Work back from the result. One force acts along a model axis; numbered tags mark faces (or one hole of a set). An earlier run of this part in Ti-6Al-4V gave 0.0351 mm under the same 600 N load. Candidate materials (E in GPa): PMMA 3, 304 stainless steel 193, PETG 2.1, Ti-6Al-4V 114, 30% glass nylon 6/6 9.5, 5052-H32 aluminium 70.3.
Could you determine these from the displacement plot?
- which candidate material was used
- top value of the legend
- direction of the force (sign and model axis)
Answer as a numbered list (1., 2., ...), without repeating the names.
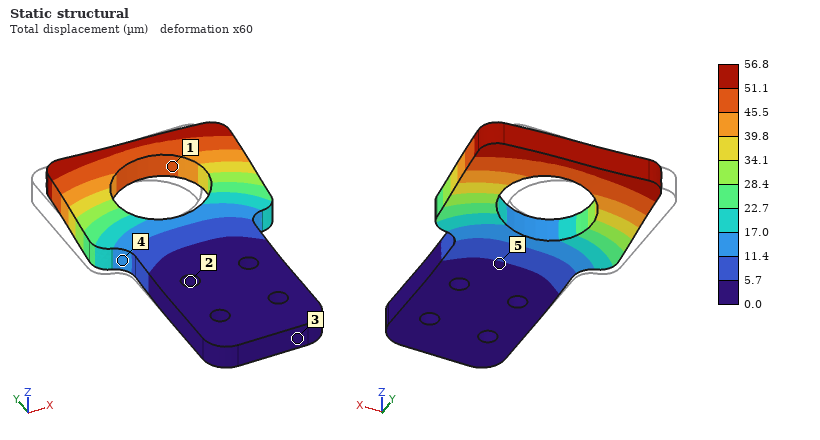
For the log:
1. 5052-H32 aluminium
2. 56.8 µm
3. +X
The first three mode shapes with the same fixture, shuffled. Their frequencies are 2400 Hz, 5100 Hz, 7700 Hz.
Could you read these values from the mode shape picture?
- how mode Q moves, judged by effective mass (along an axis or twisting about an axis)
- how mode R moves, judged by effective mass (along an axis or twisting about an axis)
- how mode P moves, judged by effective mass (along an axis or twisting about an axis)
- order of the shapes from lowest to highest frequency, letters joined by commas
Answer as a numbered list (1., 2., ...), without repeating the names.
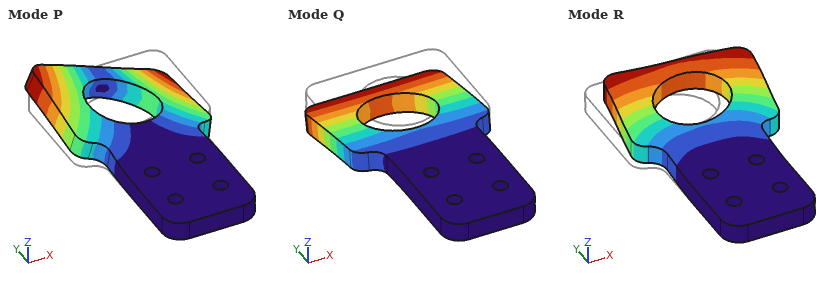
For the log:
1. along Z
2. along X
3. twisting about Y
4. Q, P, R
